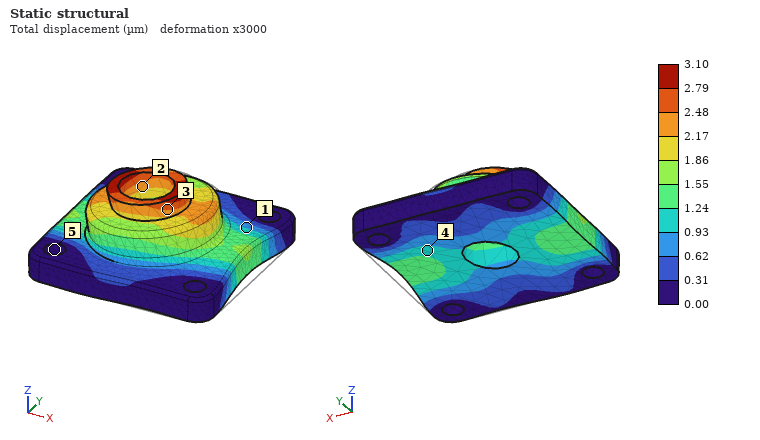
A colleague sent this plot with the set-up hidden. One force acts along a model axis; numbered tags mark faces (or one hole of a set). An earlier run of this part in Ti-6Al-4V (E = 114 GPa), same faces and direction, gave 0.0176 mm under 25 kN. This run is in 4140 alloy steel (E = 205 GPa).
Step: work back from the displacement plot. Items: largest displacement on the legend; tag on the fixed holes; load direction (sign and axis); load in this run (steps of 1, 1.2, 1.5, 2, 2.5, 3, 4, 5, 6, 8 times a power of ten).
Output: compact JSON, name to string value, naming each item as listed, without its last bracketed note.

{"largest displacement on the legend": "3.10 µm", "tag on the fixed holes": "5", "load direction": "-X", "load in this run": "8 kN"}
